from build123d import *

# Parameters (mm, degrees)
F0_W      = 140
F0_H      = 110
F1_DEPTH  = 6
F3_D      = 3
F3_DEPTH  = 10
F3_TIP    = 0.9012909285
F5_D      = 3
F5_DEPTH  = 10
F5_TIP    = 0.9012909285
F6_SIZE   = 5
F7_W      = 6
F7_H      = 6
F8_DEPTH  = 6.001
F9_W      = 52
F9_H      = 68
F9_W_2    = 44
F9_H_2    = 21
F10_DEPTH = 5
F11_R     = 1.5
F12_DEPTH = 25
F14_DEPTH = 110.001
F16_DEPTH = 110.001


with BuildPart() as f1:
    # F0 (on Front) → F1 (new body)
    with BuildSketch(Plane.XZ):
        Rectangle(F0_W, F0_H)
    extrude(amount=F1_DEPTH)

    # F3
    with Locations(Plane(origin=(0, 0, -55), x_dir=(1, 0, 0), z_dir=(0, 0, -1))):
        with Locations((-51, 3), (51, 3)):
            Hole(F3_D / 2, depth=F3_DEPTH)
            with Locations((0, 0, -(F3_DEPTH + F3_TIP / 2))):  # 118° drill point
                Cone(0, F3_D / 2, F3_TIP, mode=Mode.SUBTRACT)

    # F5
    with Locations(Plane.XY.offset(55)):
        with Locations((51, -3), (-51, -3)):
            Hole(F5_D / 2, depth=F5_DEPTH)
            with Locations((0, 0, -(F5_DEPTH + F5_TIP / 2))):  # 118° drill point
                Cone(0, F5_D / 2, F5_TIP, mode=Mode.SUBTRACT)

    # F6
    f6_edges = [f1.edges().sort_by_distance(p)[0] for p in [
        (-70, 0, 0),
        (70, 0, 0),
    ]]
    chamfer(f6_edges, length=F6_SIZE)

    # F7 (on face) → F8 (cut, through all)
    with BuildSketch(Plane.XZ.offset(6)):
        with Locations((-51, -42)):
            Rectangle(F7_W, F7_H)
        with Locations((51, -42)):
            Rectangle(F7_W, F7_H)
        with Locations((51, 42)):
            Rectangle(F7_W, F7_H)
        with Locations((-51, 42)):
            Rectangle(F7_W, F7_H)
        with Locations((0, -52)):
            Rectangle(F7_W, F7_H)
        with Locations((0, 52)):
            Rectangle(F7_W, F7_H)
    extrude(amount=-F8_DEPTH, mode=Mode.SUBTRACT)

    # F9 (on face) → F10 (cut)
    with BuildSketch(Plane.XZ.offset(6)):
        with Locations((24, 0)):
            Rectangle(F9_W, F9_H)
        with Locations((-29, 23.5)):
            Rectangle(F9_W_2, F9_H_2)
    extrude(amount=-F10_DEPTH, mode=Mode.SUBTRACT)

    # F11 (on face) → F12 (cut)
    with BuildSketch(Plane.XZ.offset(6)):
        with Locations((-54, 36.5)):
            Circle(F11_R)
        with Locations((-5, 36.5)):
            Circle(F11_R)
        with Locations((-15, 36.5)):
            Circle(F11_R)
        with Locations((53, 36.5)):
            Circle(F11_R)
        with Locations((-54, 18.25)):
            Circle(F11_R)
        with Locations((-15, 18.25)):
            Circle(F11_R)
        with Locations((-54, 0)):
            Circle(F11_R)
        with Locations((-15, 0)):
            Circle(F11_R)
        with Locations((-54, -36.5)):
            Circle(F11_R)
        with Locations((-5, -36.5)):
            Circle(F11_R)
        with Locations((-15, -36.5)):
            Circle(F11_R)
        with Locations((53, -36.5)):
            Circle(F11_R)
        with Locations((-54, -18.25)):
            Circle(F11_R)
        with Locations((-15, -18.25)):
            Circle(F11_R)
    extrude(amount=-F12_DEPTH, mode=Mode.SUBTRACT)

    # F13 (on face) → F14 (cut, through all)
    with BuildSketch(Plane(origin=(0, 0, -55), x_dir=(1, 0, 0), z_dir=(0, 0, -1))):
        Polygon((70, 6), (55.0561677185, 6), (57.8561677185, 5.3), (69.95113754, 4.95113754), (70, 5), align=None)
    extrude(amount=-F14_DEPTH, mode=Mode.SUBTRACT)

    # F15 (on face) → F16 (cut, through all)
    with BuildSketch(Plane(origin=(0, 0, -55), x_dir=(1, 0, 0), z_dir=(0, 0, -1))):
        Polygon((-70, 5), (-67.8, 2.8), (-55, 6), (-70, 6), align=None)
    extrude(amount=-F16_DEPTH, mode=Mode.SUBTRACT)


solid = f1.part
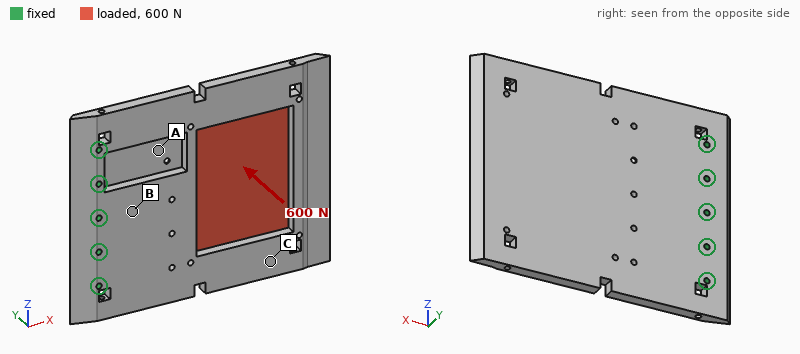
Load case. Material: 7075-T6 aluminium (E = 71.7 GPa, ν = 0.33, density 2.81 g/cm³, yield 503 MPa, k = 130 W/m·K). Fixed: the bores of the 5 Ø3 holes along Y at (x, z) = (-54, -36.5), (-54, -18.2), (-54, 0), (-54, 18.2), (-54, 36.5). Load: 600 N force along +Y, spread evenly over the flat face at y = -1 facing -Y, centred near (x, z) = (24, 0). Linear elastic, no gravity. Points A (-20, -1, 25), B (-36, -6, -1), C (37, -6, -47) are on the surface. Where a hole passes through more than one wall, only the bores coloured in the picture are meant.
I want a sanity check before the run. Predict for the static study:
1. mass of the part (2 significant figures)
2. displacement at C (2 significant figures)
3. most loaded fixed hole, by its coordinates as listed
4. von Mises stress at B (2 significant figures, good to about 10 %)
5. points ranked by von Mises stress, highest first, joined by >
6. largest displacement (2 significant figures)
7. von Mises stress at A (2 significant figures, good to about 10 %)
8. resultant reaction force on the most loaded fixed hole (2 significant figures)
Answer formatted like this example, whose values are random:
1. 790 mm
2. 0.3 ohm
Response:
1. 170 g
2. 1.2 mm
3. (-54, 18.2)
4. 62 MPa
5. B > A > C
6. 2.0 mm
7. 31 MPa
8. 850 N
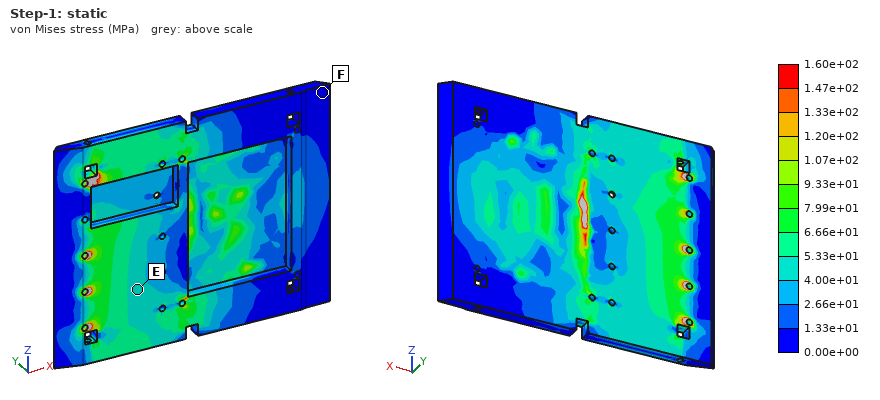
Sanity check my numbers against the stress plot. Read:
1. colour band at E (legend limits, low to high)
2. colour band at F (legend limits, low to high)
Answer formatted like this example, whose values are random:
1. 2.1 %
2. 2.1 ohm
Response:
1. 4.00e+01 to 5.33e+01 MPa
2. 0.00e+00 to 1.33e+01 MPa
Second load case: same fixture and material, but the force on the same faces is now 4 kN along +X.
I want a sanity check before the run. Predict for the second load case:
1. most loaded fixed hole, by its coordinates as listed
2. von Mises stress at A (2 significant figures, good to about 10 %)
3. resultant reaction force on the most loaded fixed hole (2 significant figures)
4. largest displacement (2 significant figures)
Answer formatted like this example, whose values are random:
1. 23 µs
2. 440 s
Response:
1. (-54, 36.5)
2. 25 MPa
3. 1.1 kN
4. 0.36 mm
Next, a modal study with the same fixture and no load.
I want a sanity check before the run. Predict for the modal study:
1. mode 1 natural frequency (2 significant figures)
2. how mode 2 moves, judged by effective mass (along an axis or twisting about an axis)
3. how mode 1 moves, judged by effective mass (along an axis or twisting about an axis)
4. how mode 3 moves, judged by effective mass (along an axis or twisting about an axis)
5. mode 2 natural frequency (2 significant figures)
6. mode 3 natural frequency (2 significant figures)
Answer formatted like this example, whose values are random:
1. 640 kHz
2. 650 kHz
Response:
1. 320 Hz
2. twisting about X
3. along Y
4. along Y
5. 650 Hz
6. 1600 Hz
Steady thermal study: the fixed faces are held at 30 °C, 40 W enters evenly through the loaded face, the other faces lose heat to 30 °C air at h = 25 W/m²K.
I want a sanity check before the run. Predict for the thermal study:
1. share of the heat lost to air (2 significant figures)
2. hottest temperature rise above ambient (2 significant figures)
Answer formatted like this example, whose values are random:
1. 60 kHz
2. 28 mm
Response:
1. 42 %
2. 52 K
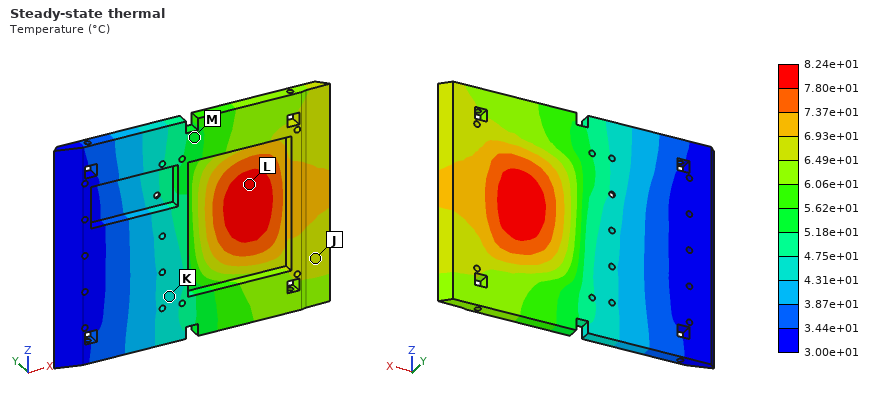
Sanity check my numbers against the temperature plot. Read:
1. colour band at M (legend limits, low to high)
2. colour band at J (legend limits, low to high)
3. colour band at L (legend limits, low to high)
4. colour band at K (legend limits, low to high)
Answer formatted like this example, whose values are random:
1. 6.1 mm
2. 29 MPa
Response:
1. 5.18e+01 to 5.62e+01 °C
2. 6.49e+01 to 6.93e+01 °C
3. 7.80e+01 to 8.24e+01 °C
4. 4.31e+01 to 4.75e+01 °C
